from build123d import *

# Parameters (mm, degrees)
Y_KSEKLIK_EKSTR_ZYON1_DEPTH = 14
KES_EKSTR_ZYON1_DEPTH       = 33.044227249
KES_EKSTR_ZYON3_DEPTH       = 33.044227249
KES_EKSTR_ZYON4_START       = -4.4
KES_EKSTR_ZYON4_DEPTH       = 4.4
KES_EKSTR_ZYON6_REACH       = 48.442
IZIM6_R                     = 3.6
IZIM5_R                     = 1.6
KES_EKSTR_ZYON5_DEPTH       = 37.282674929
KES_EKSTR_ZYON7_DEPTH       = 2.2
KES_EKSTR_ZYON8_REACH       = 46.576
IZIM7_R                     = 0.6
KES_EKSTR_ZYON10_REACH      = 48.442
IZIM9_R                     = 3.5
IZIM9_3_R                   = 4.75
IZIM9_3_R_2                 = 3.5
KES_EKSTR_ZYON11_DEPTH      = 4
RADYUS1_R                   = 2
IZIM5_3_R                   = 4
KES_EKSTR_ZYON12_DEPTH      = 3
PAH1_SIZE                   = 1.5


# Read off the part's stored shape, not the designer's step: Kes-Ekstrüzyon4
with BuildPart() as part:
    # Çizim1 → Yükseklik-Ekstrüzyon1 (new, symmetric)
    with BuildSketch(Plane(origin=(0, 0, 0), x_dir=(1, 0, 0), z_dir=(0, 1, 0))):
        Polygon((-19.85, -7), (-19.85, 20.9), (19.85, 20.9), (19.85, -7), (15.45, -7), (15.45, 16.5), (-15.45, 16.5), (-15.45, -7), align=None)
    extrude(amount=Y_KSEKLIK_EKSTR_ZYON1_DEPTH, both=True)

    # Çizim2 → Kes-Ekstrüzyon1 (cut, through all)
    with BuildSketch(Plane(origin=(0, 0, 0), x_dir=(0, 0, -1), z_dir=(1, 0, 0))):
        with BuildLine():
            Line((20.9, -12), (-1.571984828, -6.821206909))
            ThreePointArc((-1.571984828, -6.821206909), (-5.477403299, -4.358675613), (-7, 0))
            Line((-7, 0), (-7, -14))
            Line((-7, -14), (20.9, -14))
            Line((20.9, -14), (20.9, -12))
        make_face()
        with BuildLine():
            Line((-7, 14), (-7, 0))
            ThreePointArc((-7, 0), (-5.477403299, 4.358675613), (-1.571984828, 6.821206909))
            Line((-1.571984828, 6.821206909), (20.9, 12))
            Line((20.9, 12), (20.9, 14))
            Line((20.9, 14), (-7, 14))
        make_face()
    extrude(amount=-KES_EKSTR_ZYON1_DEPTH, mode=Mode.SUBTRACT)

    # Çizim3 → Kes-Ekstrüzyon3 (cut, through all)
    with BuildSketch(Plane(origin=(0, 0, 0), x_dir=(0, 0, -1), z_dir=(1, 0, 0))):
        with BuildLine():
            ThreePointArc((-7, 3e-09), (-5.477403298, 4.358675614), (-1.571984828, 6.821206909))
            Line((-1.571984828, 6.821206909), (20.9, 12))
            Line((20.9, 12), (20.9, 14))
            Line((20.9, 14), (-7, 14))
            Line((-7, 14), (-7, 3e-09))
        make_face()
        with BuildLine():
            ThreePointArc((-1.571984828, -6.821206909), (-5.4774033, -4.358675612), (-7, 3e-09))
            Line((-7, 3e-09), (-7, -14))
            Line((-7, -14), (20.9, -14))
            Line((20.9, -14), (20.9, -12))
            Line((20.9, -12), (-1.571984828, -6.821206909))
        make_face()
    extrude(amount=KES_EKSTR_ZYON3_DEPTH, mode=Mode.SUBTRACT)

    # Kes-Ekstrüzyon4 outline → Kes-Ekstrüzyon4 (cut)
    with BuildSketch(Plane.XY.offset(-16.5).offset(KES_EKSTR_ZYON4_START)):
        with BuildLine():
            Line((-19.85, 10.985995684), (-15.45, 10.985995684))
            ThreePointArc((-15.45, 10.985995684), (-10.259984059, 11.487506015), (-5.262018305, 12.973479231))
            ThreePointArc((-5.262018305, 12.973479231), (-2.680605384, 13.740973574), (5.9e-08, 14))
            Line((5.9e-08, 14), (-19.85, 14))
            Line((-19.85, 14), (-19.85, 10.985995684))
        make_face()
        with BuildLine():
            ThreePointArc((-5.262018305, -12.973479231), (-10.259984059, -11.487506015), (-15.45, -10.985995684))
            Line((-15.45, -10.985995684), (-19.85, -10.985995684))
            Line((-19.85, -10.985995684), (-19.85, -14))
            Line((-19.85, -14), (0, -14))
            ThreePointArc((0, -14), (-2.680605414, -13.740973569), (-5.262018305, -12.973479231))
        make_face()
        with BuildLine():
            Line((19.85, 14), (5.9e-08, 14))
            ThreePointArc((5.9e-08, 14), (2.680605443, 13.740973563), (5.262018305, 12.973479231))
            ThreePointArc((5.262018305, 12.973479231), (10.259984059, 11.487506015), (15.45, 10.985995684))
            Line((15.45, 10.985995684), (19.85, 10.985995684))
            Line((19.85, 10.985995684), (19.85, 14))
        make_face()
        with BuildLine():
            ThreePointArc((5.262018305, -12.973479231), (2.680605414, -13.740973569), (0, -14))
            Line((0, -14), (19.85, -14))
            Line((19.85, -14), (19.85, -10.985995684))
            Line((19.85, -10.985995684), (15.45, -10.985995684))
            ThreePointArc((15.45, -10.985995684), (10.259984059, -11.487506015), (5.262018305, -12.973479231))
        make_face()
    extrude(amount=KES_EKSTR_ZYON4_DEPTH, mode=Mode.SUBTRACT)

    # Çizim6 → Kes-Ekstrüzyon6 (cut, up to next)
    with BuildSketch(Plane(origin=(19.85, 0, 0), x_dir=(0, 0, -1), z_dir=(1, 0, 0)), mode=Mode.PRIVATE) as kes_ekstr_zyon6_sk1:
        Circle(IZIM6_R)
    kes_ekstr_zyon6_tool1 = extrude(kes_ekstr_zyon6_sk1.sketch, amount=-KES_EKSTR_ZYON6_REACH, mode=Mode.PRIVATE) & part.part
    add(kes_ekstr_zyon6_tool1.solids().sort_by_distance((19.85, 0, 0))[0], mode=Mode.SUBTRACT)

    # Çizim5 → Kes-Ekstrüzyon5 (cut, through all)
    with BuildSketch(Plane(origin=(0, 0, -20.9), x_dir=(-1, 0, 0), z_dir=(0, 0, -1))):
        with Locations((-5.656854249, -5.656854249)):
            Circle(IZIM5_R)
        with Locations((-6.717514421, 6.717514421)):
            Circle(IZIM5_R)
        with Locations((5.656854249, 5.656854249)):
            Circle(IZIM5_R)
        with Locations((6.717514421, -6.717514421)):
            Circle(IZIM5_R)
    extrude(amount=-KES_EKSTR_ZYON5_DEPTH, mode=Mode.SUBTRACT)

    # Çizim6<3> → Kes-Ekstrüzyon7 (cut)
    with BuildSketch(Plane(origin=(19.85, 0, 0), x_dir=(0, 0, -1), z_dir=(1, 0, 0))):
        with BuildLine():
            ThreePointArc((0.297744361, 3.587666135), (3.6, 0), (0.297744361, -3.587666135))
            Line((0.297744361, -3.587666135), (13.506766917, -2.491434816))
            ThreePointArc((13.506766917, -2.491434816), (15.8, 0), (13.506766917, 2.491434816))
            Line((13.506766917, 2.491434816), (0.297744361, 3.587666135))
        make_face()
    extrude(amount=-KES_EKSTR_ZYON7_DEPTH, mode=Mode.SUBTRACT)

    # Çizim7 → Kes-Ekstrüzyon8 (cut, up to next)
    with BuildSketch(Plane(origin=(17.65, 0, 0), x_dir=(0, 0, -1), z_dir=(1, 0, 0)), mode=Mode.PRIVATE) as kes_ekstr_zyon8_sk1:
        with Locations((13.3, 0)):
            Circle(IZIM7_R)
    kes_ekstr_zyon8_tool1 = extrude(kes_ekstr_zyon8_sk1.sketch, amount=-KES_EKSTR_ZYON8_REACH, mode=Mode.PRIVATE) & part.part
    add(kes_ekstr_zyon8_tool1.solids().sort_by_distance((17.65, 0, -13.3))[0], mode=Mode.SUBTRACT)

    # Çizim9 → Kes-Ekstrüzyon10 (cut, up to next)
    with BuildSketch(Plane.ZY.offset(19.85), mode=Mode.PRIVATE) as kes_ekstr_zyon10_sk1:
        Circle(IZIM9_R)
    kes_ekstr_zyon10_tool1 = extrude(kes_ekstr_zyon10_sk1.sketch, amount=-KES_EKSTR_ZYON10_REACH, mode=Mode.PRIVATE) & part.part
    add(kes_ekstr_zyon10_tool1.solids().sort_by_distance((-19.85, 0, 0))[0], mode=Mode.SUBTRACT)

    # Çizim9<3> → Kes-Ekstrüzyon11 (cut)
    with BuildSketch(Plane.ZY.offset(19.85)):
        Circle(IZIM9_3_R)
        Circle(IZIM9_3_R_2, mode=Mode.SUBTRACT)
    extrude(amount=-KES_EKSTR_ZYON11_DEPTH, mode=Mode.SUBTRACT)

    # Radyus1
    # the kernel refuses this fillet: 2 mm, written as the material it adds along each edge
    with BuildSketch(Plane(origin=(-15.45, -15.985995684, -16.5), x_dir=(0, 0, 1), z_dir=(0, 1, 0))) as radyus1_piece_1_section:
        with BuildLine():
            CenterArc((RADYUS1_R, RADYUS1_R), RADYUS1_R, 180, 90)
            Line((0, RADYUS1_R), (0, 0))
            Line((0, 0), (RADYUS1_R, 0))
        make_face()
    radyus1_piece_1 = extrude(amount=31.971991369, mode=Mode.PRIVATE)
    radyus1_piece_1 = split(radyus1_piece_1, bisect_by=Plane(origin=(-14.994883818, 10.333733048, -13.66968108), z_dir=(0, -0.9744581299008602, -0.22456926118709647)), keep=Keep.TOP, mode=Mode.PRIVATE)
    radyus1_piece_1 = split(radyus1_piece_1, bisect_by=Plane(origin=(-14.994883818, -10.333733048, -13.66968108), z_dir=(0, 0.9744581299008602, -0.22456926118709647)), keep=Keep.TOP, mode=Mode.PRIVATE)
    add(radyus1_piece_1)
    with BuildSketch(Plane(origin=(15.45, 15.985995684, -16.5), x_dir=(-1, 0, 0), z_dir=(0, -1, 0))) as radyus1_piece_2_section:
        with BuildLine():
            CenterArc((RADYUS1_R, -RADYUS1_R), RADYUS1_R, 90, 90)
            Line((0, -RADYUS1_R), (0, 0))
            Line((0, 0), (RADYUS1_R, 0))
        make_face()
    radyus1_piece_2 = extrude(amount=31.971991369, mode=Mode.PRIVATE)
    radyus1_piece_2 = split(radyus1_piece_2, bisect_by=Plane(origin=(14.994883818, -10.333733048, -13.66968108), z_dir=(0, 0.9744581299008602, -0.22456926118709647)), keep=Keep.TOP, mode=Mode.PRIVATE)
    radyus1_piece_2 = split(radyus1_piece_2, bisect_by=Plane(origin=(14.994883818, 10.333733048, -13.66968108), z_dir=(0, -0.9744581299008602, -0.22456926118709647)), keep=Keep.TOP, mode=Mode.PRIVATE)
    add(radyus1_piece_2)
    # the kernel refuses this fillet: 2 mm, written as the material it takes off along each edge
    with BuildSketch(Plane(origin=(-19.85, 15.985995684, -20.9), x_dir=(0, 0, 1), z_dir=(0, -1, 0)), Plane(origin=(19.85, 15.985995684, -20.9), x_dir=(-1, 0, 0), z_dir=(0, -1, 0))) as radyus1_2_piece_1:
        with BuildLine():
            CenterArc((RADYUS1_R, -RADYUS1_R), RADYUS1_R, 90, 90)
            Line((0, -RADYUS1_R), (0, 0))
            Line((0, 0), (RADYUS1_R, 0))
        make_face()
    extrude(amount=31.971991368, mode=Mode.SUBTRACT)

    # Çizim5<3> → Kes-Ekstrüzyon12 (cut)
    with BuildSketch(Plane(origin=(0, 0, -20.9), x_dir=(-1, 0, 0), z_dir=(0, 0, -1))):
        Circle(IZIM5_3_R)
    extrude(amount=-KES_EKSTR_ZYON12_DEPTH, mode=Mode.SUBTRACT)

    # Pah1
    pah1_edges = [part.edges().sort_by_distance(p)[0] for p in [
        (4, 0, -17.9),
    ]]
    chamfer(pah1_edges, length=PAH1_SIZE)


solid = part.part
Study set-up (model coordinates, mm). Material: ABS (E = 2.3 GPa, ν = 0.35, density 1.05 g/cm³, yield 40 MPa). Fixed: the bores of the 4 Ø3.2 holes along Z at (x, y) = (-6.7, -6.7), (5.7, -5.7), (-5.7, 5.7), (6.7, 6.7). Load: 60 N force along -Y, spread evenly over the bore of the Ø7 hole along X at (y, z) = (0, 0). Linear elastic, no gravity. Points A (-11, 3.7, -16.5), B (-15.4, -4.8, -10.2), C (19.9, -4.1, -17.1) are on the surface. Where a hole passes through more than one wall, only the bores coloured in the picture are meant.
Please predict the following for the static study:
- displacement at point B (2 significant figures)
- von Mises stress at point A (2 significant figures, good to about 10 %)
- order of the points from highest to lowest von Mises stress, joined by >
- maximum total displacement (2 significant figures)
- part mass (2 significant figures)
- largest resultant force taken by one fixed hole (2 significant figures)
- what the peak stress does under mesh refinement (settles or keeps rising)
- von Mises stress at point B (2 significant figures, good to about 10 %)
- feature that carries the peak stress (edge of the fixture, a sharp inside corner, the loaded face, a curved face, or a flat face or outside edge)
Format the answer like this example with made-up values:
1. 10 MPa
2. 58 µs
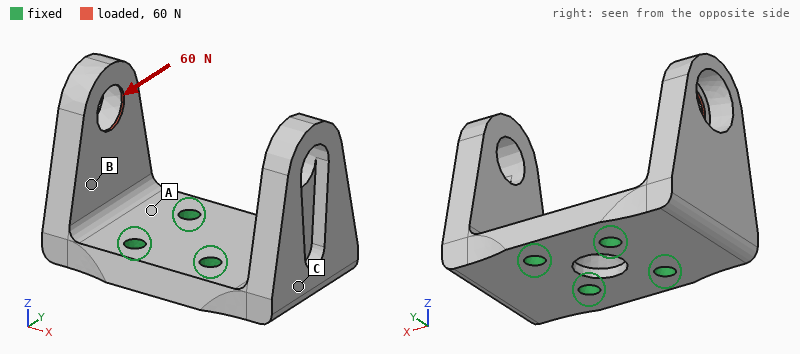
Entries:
1. 0.12 mm
2. 7.4 MPa
3. A > B > C
4. 0.38 mm
5. 6.7 g
6. 85 N
7. keeps rising
8. 4.4 MPa
9. edge of the fixture
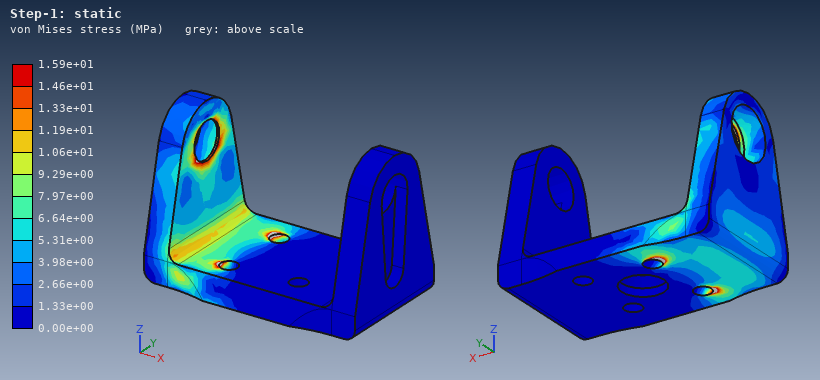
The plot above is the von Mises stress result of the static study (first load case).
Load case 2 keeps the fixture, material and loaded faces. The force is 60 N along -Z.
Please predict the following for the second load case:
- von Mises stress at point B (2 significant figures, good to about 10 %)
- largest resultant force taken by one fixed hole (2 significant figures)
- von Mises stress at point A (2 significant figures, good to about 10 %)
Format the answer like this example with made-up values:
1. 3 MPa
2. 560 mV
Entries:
1. 2.6 MPa
2. 34 N
3. 3.3 MPa
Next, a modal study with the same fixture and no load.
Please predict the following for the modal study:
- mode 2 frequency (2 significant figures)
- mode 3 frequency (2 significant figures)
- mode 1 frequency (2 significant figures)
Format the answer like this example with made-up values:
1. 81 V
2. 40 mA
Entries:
1. 1600 Hz
2. 2700 Hz
3. 1500 Hz
